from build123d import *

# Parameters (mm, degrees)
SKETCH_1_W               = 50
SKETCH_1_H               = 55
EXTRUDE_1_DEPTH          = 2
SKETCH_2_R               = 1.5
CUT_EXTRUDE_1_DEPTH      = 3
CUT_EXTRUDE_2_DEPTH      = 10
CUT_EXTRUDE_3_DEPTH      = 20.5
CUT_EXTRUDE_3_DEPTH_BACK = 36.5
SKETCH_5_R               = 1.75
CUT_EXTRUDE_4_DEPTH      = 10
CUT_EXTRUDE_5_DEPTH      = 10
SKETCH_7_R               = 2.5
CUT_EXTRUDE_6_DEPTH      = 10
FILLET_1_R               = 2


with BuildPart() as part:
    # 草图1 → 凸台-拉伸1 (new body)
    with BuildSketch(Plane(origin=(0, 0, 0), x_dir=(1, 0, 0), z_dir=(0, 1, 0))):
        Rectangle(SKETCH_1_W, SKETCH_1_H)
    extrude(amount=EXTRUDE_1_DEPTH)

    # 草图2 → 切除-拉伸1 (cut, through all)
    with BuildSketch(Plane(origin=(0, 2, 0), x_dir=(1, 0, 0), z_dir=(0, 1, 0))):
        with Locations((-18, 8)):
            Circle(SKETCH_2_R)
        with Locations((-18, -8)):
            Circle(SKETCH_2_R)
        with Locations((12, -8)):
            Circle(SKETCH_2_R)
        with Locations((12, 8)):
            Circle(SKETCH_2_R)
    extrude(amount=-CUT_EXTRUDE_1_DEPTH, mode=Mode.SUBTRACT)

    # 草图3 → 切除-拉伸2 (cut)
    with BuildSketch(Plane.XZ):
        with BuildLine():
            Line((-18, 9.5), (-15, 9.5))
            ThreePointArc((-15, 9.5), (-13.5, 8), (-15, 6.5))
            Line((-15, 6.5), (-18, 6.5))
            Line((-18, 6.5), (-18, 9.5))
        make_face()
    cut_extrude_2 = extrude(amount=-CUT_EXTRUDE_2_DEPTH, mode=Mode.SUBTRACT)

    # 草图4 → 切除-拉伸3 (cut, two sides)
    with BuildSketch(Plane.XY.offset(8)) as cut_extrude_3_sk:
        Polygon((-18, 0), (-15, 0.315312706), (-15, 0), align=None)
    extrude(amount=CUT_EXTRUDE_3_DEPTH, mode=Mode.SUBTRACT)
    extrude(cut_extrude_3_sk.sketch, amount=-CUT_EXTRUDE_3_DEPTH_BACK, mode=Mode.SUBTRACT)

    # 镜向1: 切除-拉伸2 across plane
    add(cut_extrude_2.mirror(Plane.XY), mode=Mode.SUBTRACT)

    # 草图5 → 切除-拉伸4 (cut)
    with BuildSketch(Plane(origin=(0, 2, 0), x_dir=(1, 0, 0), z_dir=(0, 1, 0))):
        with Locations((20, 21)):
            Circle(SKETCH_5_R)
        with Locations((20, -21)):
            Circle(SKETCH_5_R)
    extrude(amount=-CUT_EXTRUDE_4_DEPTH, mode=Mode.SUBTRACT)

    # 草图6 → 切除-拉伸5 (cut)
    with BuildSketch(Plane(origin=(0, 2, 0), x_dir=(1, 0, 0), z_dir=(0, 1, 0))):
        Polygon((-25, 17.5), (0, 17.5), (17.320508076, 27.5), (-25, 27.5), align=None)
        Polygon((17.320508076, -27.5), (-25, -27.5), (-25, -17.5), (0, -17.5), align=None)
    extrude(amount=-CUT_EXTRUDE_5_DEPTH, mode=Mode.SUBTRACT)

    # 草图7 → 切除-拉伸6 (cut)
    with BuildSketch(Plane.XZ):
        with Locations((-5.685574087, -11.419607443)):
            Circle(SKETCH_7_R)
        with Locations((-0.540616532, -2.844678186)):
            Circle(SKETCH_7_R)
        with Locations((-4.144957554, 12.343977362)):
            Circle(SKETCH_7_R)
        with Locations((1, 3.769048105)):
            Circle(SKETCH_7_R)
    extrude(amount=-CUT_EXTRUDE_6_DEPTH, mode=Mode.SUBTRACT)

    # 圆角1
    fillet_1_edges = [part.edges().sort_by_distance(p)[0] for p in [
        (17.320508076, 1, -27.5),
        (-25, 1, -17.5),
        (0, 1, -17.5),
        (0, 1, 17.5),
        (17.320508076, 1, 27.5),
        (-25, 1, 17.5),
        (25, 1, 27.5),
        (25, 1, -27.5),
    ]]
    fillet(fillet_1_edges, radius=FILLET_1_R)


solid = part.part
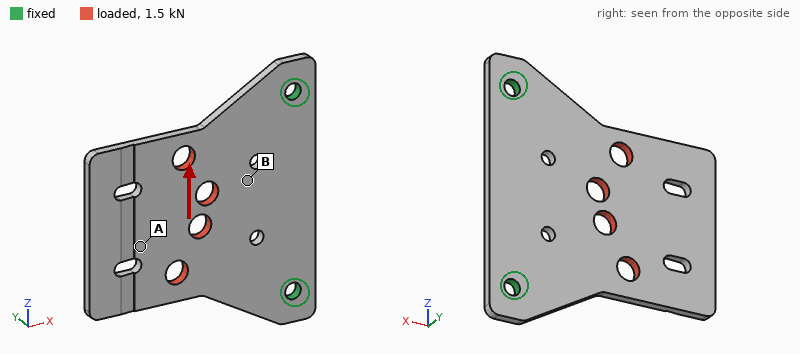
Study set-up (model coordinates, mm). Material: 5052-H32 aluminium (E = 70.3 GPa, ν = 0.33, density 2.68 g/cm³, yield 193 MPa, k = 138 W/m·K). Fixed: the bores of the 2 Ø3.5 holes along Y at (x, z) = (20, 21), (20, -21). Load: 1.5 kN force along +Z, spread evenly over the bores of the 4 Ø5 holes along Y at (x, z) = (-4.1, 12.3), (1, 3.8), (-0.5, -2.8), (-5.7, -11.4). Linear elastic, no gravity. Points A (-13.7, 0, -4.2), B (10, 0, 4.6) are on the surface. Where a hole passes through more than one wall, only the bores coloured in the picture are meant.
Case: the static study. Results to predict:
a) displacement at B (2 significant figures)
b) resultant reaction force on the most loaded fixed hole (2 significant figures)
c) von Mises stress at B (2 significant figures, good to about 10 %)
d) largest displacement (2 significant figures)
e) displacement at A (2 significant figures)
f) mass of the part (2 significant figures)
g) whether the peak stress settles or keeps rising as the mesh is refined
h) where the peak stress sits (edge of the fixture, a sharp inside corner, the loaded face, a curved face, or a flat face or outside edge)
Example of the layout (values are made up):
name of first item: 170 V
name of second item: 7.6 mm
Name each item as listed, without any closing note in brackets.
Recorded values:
displacement at B: 10 µm
resultant reaction force on the most loaded fixed hole: 1.1 kN
von Mises stress at B: 28 MPa
largest displacement: 32 µm
displacement at A: 29 µm
mass of the part: 10 g
whether the peak stress settles or keeps rising as the mesh is refined: keeps rising
where the peak stress sits: edge of the fixture
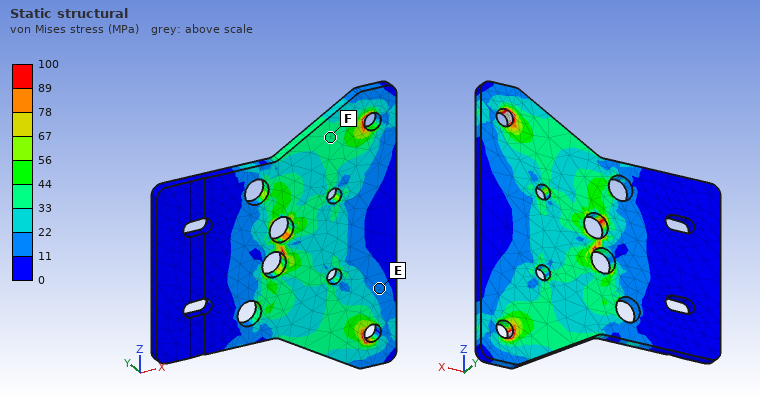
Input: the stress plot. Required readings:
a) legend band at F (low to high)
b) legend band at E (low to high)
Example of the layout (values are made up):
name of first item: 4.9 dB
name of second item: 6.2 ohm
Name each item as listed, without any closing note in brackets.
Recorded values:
legend band at F: 33 to 44 MPa
legend band at E: 11 to 22 MPa
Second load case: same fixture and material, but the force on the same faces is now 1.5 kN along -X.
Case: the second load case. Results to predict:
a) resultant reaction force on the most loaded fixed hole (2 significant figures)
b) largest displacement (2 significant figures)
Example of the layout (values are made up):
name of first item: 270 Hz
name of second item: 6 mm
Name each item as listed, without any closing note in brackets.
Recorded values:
resultant reaction force on the most loaded fixed hole: 840 N
largest displacement: 15 µm
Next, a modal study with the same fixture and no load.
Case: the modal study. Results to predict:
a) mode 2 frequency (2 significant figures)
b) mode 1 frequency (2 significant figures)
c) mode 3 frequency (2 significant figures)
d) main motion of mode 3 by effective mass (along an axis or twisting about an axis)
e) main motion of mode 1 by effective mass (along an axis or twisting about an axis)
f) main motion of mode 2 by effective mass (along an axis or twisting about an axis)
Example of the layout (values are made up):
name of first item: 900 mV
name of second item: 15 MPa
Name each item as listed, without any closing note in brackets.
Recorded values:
mode 2 frequency: 2600 Hz
mode 1 frequency: 810 Hz
mode 3 frequency: 4200 Hz
main motion of mode 3 by effective mass: along Y
main motion of mode 1 by effective mass: along Y
main motion of mode 2 by effective mass: twisting about X
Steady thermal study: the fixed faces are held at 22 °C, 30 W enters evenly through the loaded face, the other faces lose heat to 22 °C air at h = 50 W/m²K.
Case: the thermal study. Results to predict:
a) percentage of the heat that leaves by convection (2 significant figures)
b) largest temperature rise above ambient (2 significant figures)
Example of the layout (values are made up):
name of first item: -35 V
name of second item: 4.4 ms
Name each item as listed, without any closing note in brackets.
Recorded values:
percentage of the heat that leaves by convection: 29 %
largest temperature rise above ambient: 68 K
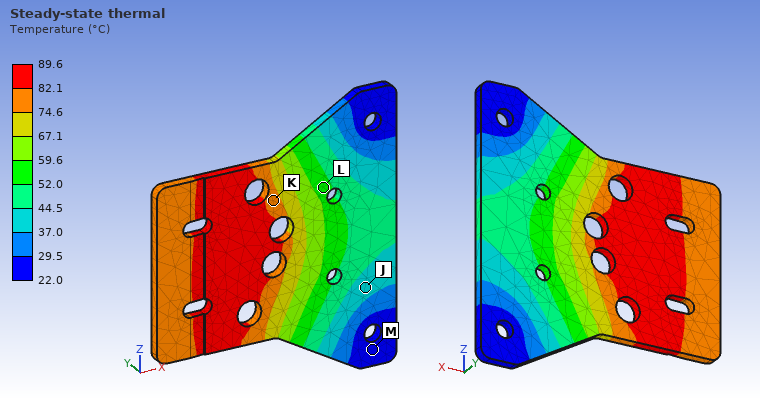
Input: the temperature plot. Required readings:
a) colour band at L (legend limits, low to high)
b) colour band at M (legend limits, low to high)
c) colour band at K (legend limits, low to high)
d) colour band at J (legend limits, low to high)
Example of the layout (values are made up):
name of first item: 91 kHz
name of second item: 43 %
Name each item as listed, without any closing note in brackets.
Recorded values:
colour band at L: 52.0 to 59.6 °C
colour band at M: 22.0 to 29.5 °C
colour band at K: 74.6 to 82.1 °C
colour band at J: 37.0 to 44.5 °C
